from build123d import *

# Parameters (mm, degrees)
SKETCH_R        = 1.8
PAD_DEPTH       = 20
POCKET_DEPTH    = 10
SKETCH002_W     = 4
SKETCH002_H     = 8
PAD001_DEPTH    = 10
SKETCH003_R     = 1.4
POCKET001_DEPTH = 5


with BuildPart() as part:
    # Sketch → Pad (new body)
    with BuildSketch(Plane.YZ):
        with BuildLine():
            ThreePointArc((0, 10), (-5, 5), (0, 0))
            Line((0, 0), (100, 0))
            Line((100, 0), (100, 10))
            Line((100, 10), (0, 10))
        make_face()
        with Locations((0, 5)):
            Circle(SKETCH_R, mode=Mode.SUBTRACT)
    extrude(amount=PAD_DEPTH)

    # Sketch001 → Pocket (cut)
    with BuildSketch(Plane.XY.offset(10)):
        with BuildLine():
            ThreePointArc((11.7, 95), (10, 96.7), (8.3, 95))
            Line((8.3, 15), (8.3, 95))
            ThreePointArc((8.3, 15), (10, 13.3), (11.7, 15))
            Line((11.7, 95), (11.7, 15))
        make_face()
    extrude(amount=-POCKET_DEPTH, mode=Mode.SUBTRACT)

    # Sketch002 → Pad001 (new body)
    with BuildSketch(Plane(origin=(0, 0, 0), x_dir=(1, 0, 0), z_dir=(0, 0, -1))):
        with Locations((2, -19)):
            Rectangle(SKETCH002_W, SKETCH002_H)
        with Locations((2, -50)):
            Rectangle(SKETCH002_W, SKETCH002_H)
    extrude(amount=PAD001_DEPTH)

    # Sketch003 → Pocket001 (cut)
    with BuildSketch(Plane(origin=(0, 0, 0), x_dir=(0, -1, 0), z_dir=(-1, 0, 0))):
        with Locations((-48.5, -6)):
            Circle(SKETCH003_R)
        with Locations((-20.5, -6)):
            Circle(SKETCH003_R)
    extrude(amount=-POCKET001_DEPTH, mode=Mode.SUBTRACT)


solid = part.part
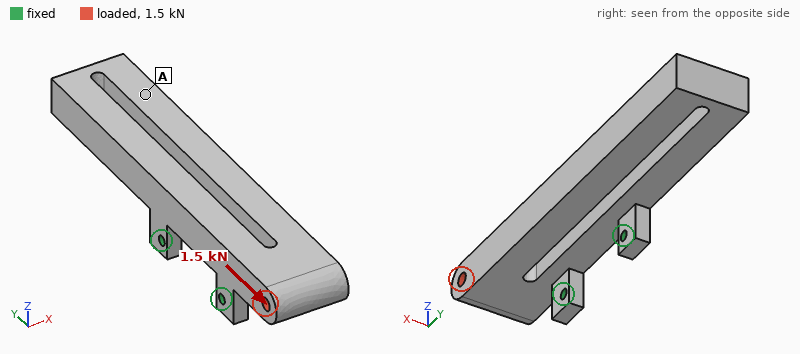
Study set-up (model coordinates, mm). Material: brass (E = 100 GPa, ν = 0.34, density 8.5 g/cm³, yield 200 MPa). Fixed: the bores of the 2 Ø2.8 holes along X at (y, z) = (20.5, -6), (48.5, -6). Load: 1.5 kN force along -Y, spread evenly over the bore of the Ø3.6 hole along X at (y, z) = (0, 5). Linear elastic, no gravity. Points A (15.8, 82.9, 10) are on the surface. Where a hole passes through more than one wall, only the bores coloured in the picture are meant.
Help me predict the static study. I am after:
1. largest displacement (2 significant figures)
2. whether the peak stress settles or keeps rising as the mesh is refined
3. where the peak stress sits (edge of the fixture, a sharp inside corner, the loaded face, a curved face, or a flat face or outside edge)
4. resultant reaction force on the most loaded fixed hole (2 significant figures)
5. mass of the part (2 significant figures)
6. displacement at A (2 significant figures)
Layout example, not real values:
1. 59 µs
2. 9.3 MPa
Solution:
1. 0.12 mm
2. keeps rising
3. edge of the fixture
4. 940 N
5. 160 g
6. 0.088 mm
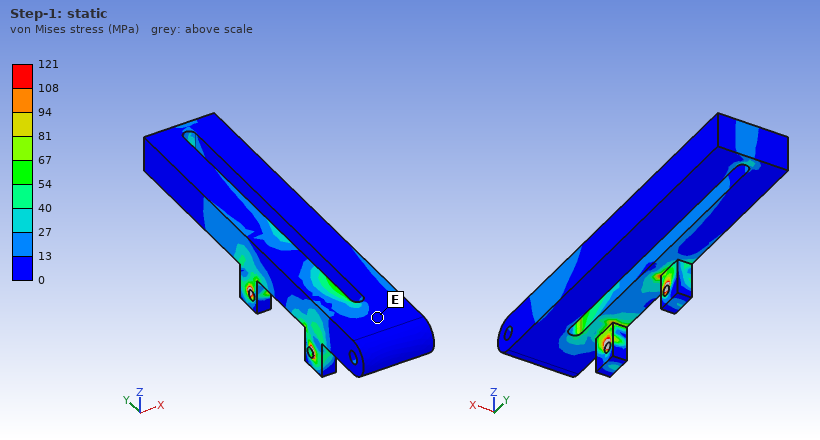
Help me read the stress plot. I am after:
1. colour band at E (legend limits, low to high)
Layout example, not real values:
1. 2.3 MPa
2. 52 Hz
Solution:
1. 0 to 13 MPa
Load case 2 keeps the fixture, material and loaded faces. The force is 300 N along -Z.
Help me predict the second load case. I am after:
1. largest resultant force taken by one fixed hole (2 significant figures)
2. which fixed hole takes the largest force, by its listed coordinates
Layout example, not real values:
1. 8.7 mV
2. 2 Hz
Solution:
1. 490 N
2. (20.5, -6)
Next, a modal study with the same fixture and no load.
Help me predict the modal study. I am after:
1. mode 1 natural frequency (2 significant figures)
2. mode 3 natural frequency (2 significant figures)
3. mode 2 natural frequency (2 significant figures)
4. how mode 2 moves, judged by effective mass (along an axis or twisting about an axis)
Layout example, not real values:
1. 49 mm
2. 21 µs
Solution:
1. 810 Hz
2. 1500 Hz
3. 1000 Hz
4. along Z
